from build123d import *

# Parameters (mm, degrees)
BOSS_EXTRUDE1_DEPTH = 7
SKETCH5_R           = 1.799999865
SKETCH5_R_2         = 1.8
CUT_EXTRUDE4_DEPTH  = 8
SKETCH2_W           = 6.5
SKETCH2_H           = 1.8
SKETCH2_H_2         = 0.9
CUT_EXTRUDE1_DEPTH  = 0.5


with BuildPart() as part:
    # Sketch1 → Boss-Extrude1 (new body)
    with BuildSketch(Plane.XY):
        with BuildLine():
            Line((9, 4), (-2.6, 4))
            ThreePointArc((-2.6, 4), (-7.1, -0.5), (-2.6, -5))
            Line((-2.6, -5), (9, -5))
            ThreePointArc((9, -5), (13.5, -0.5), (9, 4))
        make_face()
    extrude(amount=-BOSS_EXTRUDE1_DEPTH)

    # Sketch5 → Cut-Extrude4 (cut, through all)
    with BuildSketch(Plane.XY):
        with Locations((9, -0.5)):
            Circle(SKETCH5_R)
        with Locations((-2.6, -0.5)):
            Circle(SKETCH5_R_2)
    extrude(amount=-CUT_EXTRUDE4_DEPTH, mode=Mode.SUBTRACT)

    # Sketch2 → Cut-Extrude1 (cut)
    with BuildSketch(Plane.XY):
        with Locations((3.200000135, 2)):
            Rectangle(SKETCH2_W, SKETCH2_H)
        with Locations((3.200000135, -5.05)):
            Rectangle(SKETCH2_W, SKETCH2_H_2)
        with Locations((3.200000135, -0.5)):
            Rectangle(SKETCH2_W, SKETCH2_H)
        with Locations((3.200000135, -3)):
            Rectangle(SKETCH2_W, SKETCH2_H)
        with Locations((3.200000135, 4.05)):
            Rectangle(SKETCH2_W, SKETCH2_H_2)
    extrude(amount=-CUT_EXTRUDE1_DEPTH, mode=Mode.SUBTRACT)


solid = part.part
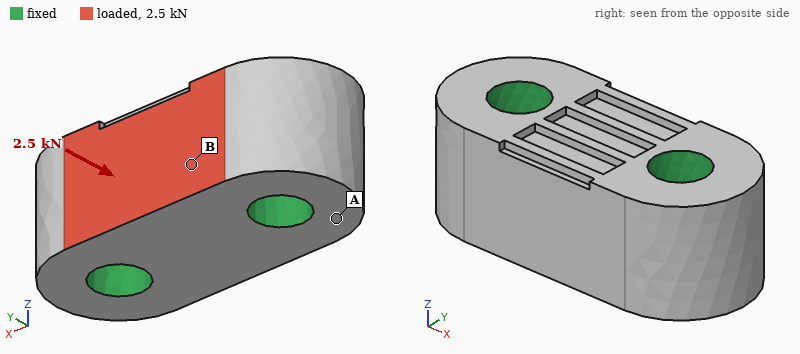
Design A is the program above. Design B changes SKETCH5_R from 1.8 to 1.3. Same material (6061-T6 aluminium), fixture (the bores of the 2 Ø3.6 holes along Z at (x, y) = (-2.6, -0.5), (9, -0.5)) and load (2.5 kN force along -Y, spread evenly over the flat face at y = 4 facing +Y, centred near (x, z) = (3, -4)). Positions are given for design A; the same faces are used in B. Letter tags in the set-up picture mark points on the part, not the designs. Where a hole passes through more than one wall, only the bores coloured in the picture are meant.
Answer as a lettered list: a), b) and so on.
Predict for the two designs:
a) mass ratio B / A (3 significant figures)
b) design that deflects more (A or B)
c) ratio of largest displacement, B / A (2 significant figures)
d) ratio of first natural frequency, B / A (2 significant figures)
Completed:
a) 1.03
b) B
c) 1.1
d) 0.92
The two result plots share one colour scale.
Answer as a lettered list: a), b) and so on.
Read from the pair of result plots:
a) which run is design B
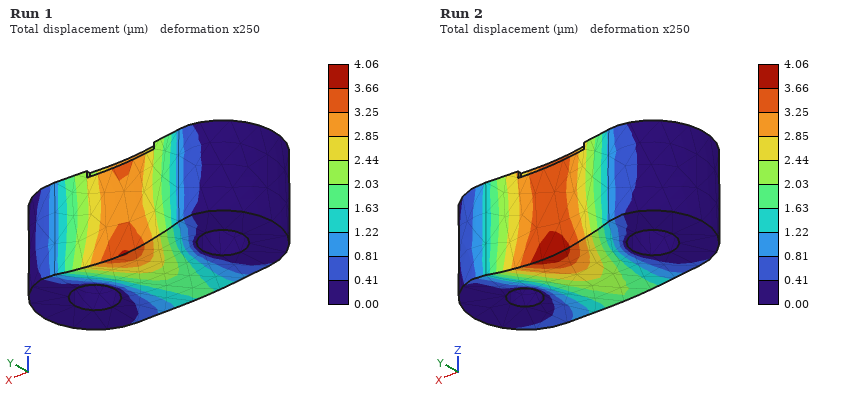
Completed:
a) Run 2
